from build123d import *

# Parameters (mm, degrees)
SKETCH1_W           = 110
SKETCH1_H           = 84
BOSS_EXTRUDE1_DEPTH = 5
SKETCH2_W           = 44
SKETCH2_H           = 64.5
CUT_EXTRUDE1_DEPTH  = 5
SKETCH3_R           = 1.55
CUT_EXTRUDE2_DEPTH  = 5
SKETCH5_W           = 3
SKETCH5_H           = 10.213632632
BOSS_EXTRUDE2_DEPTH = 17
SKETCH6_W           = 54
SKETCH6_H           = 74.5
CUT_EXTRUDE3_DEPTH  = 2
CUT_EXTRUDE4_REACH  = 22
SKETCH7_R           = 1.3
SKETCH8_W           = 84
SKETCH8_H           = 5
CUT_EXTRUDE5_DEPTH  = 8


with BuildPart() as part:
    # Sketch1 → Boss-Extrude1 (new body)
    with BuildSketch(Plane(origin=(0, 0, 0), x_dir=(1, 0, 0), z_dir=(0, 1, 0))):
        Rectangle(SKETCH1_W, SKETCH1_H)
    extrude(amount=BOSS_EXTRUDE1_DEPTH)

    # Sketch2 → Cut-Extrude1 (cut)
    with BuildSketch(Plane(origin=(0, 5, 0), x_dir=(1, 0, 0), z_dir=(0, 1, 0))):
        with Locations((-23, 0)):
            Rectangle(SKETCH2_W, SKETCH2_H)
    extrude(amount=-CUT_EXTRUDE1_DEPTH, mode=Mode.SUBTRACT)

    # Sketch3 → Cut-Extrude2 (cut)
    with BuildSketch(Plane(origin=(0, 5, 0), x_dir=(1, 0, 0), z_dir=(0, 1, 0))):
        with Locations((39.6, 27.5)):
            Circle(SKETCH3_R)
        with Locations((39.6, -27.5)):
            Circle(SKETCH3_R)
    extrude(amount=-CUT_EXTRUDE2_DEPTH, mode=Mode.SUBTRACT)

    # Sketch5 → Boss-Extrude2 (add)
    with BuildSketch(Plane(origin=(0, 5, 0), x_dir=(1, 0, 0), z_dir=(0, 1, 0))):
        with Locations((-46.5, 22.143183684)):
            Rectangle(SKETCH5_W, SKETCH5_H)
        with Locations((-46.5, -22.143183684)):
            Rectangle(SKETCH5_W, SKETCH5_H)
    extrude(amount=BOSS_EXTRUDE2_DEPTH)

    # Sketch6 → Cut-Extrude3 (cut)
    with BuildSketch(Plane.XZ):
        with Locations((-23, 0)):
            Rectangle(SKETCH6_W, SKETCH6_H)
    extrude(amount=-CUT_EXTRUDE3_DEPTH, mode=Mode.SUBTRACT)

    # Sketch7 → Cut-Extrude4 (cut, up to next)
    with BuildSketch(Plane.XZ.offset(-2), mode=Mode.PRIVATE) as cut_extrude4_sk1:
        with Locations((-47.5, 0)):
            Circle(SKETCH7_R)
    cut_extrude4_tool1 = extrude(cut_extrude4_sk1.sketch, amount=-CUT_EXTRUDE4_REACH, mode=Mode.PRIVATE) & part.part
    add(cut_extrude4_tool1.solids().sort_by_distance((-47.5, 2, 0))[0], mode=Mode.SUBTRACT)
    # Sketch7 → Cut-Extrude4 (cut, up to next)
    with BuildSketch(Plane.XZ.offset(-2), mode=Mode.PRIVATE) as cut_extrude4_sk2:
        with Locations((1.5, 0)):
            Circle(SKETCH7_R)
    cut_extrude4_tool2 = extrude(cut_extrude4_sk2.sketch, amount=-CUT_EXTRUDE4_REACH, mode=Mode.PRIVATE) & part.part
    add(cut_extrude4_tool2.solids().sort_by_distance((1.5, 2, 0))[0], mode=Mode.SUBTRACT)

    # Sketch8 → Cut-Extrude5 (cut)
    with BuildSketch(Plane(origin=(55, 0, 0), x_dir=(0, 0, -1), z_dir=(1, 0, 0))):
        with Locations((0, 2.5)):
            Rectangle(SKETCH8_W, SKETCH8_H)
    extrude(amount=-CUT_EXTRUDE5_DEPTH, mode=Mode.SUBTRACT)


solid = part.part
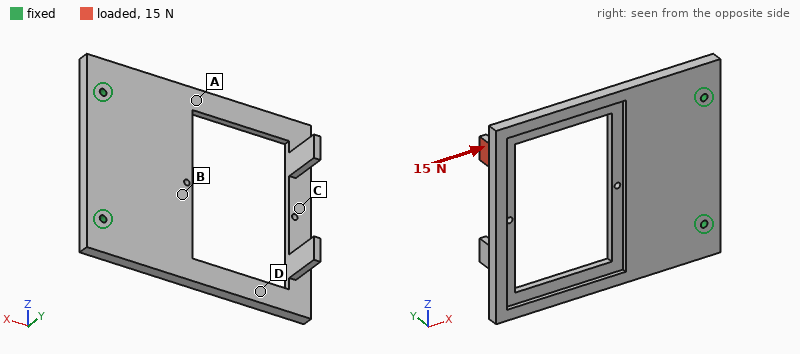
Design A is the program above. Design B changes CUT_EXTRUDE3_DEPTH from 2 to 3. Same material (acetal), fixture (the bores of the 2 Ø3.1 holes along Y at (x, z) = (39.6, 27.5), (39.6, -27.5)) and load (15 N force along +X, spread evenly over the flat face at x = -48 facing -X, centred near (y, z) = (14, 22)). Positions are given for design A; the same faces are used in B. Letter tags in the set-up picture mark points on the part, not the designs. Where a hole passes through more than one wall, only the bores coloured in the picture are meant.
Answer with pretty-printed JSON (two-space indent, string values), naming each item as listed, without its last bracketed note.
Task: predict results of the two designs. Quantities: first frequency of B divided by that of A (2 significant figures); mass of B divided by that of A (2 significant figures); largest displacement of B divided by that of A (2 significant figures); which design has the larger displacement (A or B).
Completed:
{
  "first frequency of B divided by that of A": "1.0",
  "mass of B divided by that of A": "0.96",
  "largest displacement of B divided by that of A": "1.1",
  "which design has the larger displacement": "B"
}
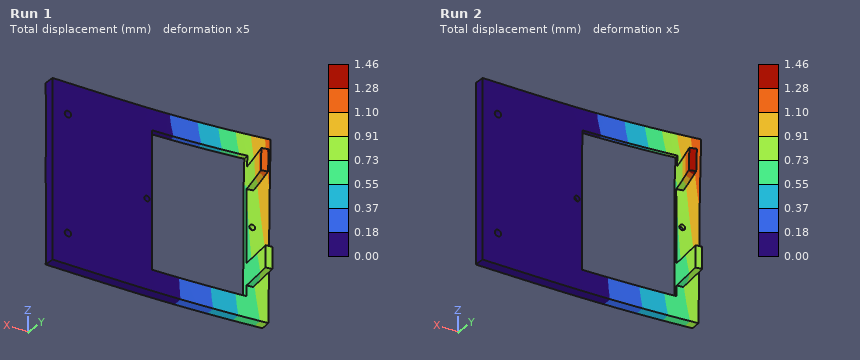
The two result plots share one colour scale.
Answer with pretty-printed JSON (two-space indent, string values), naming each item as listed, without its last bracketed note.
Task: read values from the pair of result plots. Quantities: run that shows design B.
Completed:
{
  "run that shows design B": "Run 2"
}
